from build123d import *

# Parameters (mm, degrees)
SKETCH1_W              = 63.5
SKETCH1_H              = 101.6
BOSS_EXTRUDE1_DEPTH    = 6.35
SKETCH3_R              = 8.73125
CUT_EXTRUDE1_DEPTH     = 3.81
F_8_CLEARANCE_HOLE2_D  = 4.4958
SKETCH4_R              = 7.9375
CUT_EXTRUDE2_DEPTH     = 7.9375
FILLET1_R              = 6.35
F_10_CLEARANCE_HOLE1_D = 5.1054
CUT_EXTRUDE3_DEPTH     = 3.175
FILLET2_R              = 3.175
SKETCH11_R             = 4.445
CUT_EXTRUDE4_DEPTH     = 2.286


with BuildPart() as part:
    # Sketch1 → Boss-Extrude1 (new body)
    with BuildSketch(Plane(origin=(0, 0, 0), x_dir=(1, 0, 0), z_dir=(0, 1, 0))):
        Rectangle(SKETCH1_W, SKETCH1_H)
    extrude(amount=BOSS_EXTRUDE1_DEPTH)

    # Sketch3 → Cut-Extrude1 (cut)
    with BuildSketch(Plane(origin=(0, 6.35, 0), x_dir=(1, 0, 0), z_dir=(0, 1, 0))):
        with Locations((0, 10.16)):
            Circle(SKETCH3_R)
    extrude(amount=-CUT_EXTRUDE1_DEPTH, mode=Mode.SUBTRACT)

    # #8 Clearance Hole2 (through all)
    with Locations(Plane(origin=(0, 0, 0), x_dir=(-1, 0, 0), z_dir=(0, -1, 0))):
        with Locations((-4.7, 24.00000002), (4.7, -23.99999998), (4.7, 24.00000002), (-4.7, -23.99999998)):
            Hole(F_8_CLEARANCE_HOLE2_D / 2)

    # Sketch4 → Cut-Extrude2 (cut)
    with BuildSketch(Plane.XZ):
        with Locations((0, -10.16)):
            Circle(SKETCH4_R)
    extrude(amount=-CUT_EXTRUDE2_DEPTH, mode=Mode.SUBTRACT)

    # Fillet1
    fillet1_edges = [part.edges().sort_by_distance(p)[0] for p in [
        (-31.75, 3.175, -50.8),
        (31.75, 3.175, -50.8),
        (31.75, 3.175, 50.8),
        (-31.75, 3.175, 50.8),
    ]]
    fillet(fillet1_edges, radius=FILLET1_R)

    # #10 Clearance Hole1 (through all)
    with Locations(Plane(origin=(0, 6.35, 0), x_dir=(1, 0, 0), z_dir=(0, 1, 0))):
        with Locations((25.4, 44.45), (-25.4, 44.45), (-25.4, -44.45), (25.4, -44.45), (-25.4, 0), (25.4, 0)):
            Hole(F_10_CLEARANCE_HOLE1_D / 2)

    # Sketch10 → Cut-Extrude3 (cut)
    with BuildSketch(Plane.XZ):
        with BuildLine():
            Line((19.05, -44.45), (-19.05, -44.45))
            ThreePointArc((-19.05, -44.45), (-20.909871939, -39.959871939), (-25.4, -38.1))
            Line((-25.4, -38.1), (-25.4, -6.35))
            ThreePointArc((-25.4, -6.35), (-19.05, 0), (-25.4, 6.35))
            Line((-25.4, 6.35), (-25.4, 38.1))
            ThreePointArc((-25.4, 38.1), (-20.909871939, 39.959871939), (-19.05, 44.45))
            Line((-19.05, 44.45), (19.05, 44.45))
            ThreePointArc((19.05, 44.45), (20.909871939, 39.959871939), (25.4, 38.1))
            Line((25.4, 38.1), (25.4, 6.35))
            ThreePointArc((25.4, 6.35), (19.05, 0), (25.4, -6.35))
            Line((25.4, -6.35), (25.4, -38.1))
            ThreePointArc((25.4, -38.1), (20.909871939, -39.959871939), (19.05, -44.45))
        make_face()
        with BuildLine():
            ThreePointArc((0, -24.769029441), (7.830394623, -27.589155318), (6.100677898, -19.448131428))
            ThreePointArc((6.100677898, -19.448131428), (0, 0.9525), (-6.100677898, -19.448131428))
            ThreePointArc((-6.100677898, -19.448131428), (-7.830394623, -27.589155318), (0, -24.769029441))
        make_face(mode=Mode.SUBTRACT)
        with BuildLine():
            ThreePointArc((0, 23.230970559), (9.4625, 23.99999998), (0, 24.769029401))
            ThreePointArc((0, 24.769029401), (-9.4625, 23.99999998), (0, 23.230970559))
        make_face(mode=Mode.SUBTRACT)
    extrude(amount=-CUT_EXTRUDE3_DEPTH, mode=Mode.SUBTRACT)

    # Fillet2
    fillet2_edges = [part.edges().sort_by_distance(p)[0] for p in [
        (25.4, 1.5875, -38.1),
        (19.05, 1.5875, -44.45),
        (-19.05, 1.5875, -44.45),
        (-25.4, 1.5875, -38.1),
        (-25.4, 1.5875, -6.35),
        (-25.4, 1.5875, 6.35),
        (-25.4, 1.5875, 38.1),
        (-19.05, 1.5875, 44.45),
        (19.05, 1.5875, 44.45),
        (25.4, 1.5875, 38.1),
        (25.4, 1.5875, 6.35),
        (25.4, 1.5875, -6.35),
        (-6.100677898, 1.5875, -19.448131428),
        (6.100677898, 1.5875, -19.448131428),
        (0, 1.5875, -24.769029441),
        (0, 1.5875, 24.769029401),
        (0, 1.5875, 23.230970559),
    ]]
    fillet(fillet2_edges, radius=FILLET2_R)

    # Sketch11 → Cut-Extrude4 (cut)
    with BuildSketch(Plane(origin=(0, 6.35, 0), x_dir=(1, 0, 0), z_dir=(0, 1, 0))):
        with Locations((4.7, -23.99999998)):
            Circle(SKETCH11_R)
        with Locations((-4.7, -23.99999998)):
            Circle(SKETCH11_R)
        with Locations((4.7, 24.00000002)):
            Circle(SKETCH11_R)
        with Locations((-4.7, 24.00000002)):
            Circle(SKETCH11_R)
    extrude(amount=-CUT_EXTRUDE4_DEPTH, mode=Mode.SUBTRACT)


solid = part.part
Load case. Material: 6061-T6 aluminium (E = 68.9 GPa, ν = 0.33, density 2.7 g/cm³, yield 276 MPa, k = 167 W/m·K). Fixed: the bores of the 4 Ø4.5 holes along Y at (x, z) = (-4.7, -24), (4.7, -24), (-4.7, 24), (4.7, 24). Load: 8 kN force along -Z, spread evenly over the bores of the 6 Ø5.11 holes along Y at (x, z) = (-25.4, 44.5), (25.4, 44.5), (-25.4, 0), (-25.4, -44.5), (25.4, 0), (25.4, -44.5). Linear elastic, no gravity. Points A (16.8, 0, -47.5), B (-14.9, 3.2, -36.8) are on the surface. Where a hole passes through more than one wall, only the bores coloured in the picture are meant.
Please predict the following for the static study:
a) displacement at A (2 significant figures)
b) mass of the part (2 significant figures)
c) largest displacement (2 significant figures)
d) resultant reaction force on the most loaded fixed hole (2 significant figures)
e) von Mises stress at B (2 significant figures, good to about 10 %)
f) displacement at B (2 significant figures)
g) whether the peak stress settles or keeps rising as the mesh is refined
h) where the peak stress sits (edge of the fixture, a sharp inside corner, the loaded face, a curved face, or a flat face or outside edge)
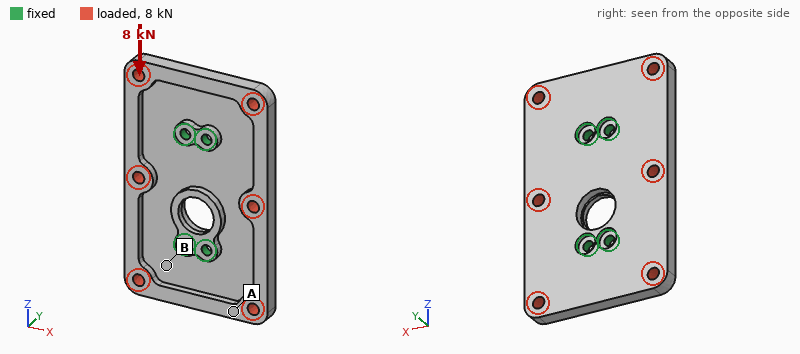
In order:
35 µm
71 g
56 µm
2.1 kN
31 MPa
16 µm
keeps rising
edge of the fixture
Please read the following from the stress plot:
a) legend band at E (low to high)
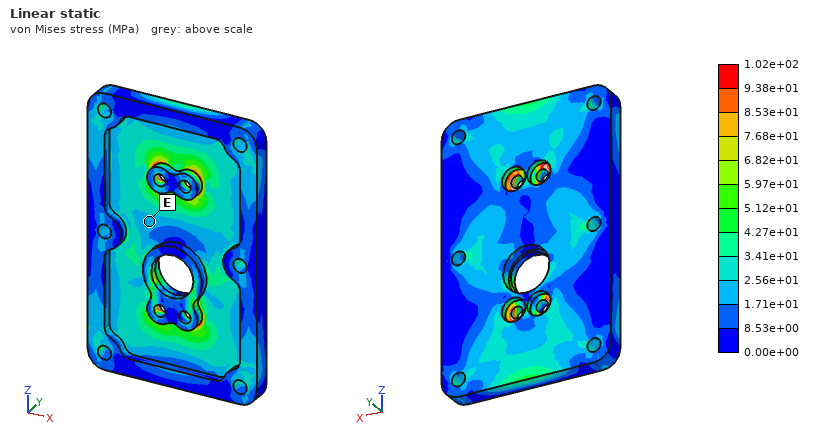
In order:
1.71e+01 to 2.56e+01 MPa
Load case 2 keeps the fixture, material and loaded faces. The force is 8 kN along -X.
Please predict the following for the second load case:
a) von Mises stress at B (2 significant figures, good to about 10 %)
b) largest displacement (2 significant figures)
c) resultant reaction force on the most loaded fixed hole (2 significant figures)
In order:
39 MPa
99 µm
2.0 kN
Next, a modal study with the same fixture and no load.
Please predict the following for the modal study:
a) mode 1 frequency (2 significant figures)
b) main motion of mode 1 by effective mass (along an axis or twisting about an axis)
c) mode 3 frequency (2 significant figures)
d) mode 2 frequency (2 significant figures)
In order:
2200 Hz
twisting about Z
2700 Hz
2600 Hz
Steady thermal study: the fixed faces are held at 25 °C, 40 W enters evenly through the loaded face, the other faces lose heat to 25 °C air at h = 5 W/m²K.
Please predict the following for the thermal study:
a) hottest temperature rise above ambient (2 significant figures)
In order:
18 K
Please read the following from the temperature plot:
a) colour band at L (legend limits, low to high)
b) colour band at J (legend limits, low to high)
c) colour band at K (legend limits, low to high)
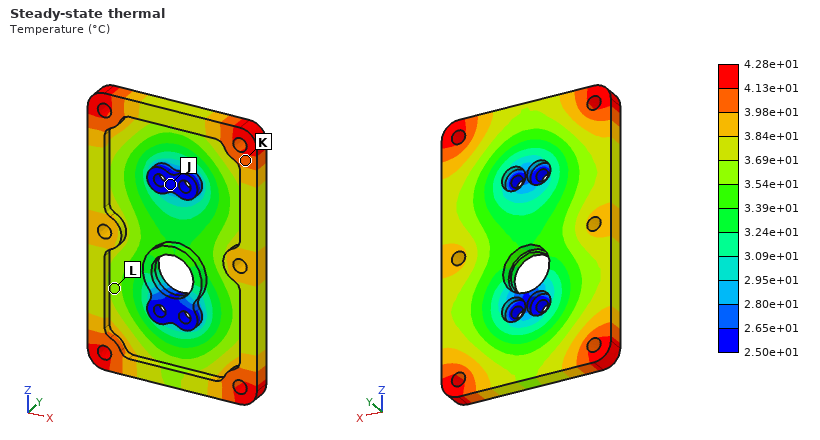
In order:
3.54e+01 to 3.69e+01 °C
2.50e+01 to 2.65e+01 °C
3.98e+01 to 4.13e+01 °C
